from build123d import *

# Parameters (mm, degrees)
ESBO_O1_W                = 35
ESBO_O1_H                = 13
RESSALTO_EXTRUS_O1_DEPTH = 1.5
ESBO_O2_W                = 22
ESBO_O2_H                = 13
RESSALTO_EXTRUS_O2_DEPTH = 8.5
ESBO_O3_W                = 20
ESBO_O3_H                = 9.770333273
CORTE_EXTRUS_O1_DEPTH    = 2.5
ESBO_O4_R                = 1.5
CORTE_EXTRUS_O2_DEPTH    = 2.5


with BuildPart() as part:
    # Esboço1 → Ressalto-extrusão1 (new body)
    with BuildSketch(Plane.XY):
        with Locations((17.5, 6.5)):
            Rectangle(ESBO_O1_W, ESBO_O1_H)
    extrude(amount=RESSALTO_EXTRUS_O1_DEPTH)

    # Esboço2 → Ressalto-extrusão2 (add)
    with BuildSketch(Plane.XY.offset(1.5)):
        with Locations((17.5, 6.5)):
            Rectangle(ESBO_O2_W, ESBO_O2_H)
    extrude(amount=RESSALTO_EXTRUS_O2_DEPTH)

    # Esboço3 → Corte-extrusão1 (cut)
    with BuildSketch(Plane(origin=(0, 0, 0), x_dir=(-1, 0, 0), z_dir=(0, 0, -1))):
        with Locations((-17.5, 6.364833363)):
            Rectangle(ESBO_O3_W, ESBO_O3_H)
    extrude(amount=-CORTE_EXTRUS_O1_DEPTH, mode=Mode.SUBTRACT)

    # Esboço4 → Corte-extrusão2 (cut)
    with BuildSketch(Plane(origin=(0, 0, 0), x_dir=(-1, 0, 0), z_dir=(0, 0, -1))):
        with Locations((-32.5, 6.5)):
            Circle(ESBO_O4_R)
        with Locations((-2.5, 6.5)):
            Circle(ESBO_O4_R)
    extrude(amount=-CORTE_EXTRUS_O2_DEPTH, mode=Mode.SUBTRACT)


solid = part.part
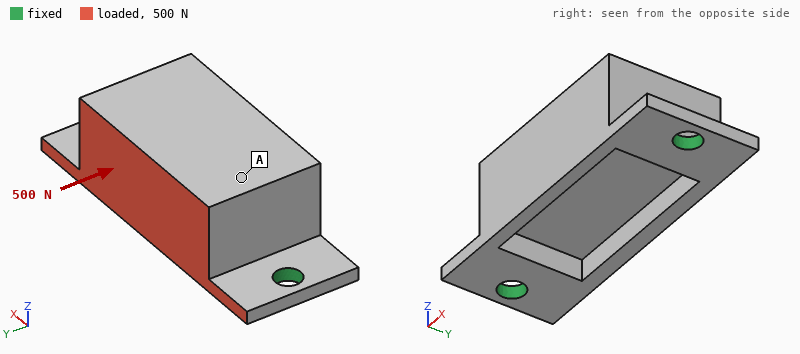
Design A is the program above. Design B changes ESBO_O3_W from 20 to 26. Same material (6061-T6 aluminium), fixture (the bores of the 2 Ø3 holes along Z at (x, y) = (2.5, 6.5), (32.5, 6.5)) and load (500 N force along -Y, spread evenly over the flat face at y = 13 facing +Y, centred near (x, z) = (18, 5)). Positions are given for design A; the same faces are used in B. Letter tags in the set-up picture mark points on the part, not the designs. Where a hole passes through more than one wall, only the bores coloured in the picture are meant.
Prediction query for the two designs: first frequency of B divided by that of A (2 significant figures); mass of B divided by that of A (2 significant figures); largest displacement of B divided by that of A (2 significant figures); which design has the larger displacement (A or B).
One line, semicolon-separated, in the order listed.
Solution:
0.70; 0.96; 2.1; B
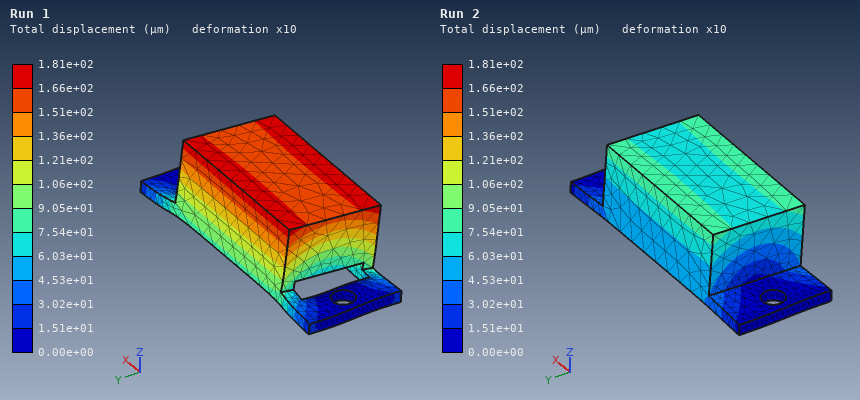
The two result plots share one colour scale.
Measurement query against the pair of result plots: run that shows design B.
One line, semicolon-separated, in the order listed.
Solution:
Run 1
